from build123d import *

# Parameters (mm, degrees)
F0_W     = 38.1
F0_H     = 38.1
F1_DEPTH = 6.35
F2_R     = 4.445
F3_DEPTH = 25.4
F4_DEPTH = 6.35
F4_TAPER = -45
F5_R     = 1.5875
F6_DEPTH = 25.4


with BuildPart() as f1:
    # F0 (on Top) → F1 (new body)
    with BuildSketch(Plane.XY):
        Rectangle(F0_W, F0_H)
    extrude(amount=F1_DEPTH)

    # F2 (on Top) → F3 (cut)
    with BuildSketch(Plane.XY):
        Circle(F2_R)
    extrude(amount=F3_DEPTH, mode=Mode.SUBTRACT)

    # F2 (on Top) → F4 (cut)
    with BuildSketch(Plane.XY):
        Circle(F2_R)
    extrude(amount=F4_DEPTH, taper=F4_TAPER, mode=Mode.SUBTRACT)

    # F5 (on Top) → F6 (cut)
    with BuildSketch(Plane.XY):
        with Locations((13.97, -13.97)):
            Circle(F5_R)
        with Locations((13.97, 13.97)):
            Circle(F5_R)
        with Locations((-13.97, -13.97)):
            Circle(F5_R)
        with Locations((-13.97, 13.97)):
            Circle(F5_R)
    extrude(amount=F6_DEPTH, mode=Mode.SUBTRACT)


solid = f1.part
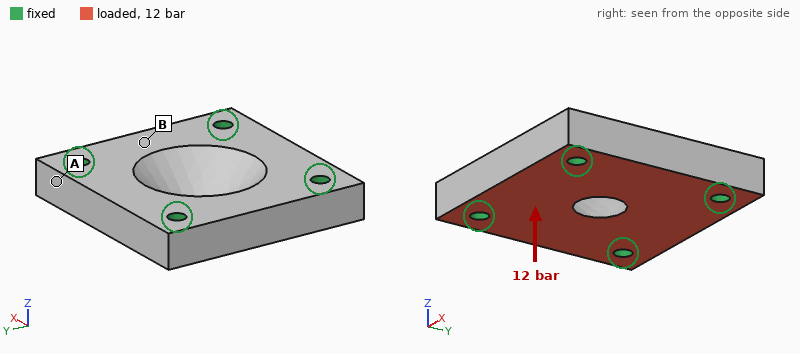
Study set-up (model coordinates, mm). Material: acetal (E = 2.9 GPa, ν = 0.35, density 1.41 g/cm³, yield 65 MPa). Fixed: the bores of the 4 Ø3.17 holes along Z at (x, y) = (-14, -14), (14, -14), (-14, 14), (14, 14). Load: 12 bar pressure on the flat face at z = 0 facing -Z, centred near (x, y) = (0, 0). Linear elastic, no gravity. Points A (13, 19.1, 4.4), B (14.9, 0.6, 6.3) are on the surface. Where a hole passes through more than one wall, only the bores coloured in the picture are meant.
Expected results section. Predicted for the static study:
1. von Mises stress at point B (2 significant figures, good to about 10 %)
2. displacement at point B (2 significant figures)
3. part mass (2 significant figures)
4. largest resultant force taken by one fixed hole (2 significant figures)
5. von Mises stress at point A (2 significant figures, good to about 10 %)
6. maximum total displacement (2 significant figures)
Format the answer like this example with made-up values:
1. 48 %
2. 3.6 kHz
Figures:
1. 7.9 MPa
2. 0.064 mm
3. 11 g
4. 410 N
5. 3.3 MPa
6. 0.14 mm
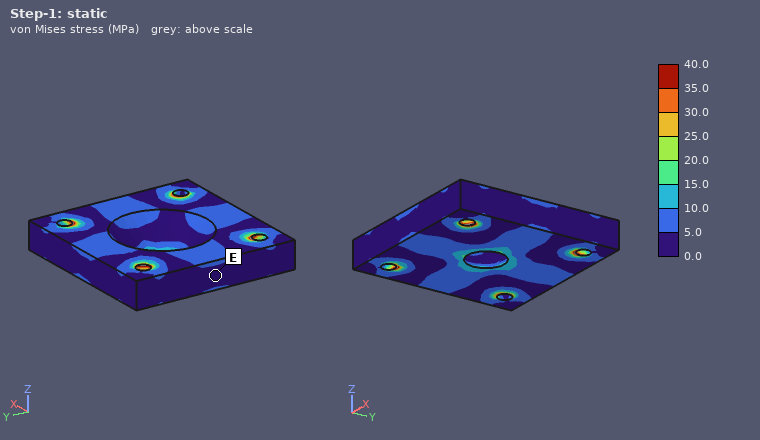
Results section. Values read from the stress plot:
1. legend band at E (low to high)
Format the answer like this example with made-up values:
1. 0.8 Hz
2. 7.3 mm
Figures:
1. 0.0 to 5.0 MPa
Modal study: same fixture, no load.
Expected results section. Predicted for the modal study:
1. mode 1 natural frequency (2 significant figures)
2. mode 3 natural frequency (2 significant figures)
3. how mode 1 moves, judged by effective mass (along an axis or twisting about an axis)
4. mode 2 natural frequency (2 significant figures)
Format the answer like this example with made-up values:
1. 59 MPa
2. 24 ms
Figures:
1. 7800 Hz
2. 9700 Hz
3. along Z
4. 9700 Hz
